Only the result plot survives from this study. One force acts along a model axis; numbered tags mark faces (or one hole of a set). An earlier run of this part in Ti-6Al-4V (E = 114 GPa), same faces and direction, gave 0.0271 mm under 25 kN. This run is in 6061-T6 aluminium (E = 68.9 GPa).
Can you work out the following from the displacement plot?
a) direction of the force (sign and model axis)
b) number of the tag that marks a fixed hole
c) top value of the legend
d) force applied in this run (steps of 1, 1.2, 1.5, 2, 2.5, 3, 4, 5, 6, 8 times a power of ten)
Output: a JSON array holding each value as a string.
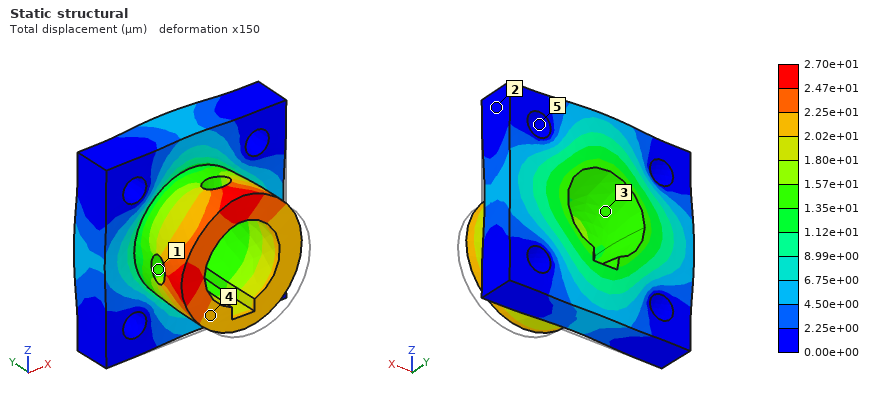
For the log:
["+Y", "5", "2.70e+01 µm", "15 kN"]
